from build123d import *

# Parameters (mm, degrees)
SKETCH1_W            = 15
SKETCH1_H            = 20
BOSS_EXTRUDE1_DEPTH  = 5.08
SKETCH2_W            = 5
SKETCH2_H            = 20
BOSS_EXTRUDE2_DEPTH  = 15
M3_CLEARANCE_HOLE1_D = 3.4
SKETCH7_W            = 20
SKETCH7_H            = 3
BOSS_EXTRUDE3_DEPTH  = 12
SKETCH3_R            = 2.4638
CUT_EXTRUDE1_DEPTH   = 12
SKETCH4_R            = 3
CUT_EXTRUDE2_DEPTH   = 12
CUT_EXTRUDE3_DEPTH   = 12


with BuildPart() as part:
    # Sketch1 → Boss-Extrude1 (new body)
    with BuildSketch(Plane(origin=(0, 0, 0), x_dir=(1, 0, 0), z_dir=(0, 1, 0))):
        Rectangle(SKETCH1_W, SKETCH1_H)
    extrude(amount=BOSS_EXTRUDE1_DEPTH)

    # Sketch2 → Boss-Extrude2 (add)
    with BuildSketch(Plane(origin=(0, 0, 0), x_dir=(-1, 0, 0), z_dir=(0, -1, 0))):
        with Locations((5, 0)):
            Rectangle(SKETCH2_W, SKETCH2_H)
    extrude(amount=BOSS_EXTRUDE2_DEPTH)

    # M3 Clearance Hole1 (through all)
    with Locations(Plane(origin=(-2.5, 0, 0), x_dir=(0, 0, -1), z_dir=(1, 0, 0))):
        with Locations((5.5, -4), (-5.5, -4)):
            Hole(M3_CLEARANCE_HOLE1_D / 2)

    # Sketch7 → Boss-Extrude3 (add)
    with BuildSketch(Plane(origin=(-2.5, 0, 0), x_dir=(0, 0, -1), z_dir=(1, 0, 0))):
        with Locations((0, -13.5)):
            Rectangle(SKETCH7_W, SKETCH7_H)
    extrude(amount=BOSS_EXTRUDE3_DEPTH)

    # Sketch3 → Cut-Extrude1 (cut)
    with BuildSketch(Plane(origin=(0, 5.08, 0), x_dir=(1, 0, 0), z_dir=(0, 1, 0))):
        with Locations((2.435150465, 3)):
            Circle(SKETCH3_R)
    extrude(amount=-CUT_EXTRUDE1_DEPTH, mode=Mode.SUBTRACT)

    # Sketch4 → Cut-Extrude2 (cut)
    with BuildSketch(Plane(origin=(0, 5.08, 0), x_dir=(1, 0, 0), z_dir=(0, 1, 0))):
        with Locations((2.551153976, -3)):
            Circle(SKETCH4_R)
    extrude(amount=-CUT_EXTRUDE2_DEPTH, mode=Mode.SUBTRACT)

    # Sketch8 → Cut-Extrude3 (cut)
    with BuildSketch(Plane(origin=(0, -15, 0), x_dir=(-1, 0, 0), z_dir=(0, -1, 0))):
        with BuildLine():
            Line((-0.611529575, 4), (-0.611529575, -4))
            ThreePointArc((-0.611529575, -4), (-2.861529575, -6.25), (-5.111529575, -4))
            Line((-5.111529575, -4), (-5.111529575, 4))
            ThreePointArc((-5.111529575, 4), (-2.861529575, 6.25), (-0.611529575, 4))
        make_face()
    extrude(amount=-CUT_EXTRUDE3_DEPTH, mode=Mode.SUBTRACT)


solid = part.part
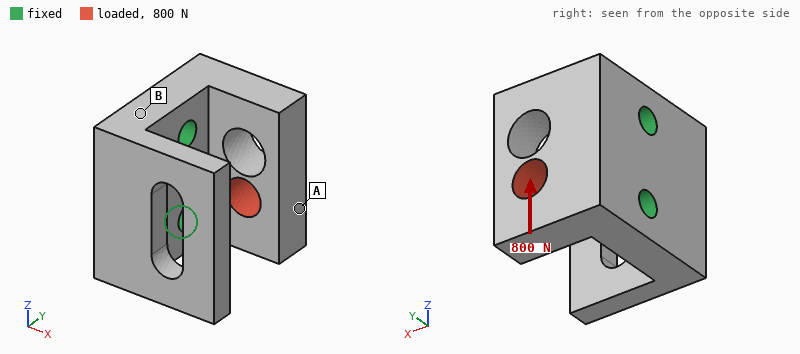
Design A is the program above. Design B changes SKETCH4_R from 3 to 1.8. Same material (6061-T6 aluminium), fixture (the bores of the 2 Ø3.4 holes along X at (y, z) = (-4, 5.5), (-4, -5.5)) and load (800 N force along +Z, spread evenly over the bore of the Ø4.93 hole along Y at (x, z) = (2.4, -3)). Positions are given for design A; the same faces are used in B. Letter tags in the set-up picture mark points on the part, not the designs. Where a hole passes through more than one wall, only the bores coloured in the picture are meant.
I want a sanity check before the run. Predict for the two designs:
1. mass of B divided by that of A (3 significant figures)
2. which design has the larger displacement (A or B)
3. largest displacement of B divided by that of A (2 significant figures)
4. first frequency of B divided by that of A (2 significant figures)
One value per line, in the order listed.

1.03
A
0.75
1.0
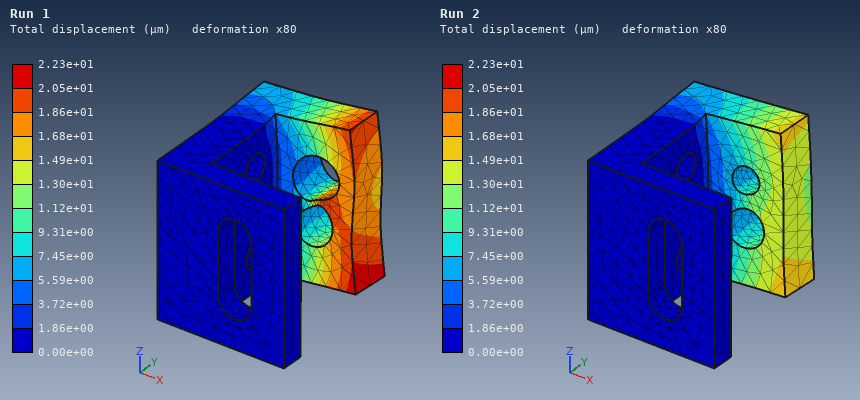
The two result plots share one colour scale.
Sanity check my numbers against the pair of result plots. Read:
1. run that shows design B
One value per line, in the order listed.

Run 2
